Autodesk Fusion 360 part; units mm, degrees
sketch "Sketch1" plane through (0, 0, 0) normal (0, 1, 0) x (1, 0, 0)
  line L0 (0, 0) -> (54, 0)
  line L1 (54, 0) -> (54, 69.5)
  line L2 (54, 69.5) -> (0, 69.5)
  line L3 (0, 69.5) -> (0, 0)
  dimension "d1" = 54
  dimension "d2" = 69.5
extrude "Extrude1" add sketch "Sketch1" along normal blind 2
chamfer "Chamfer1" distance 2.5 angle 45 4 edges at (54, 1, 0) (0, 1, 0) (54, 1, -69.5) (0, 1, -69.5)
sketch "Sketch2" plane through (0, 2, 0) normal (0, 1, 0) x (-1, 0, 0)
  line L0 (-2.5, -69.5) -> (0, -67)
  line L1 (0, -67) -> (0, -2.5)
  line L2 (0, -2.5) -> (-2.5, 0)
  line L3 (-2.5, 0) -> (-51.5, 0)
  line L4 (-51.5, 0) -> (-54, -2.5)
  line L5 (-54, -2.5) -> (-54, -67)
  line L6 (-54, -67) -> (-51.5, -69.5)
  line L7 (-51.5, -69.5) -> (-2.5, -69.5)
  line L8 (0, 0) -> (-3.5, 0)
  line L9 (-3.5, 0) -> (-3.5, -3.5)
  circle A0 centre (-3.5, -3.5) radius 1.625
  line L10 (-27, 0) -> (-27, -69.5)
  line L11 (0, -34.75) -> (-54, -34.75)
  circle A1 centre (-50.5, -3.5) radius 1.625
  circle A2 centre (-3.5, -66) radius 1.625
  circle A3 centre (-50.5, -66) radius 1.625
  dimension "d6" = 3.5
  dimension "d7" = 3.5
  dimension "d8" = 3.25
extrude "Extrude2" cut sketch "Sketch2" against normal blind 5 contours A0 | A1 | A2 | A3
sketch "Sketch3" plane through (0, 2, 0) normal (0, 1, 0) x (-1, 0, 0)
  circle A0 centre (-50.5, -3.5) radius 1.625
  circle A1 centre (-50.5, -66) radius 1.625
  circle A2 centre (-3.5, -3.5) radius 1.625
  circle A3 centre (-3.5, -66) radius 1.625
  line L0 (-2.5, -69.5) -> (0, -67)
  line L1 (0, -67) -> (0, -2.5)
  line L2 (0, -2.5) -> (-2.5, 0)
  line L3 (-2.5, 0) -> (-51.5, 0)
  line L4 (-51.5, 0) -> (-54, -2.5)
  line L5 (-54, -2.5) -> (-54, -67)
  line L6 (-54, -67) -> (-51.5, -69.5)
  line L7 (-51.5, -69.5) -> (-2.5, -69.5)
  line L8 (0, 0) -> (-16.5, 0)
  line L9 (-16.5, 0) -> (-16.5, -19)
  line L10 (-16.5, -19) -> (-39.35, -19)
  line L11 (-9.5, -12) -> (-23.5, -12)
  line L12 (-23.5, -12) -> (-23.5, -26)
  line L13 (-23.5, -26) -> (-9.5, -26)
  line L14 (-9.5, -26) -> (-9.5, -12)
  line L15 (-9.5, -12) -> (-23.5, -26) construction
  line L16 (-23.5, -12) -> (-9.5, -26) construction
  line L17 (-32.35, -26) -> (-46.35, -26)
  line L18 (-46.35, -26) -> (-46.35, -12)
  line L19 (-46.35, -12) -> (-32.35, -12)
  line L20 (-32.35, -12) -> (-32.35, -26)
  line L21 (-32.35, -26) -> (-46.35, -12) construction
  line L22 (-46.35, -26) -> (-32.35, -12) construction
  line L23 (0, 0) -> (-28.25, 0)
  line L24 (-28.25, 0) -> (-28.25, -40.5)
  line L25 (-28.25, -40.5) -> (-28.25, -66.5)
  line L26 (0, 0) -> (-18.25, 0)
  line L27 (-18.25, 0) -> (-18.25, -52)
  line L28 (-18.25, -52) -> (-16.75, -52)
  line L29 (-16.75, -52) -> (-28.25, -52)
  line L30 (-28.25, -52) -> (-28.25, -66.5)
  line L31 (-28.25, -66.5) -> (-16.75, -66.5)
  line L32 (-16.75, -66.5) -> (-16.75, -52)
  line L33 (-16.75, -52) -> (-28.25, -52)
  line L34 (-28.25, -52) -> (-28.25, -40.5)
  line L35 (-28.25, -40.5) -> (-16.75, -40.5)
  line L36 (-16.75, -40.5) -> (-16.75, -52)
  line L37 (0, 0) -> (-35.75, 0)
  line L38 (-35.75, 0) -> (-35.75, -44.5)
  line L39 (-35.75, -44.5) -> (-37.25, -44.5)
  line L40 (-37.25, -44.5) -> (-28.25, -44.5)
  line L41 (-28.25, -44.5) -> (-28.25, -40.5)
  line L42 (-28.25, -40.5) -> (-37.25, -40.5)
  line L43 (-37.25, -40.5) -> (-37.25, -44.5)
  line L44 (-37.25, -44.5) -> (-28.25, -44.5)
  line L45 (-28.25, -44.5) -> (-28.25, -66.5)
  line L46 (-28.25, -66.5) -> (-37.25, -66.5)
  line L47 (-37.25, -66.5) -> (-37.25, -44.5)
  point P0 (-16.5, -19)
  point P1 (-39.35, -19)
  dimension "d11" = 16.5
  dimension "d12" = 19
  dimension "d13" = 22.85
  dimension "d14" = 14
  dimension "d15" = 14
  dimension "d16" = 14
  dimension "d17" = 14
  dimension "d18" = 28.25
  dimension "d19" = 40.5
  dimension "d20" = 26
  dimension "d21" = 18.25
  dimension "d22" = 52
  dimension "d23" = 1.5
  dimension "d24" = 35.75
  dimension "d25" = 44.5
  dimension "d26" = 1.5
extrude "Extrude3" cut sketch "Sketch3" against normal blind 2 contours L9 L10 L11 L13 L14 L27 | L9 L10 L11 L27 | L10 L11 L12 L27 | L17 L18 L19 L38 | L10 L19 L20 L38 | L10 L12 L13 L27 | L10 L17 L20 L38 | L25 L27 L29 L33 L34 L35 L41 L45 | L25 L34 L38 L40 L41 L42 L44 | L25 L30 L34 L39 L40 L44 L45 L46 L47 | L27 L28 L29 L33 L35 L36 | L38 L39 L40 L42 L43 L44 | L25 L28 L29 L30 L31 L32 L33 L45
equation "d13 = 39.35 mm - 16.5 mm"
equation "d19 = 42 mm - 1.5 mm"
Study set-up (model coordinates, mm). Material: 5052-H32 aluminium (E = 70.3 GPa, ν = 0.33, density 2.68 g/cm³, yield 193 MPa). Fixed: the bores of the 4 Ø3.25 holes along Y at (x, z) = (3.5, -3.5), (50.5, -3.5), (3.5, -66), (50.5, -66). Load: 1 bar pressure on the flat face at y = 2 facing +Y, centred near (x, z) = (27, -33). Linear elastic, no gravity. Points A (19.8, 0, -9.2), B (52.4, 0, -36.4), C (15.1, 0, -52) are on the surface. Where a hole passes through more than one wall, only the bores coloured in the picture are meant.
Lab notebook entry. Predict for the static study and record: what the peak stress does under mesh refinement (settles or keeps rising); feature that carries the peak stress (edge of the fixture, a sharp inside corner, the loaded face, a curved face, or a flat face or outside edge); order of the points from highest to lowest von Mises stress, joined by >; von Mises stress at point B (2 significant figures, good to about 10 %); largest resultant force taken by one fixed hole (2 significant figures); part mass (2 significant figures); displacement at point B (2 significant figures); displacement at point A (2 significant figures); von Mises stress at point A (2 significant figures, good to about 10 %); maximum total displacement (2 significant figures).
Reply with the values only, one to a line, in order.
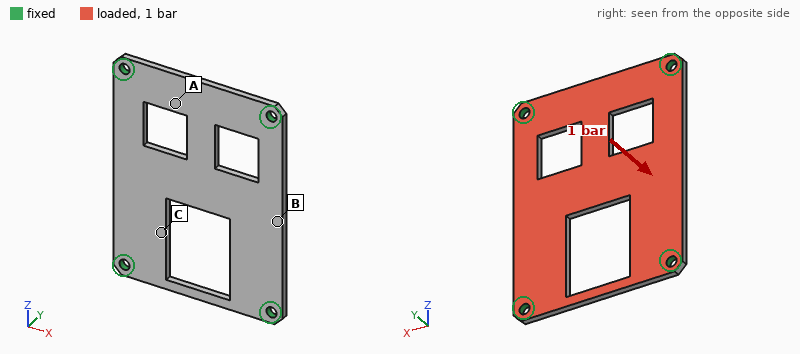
keeps rising
edge of the fixture
B > A > C
29 MPa
73 N
15 g
0.10 mm
0.052 mm
18 MPa
0.15 mm
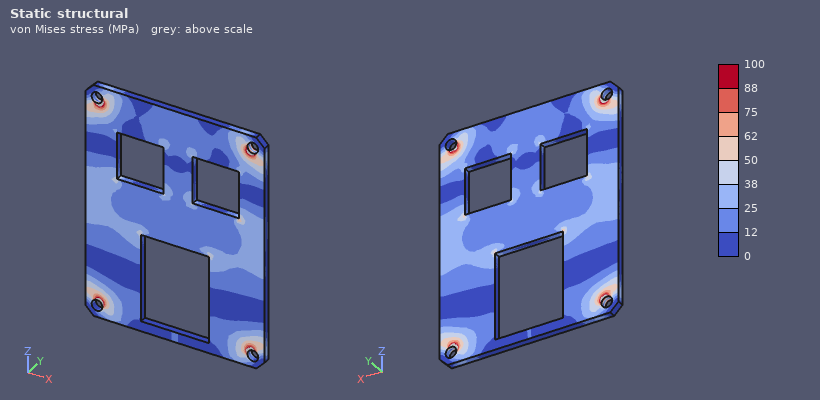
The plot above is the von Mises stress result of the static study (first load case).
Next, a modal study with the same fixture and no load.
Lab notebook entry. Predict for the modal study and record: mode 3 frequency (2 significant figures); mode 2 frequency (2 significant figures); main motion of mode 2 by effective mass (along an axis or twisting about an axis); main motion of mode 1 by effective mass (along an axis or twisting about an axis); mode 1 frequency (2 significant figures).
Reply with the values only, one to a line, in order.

4500 Hz
3100 Hz
twisting about Z
along Y
2100 Hz
